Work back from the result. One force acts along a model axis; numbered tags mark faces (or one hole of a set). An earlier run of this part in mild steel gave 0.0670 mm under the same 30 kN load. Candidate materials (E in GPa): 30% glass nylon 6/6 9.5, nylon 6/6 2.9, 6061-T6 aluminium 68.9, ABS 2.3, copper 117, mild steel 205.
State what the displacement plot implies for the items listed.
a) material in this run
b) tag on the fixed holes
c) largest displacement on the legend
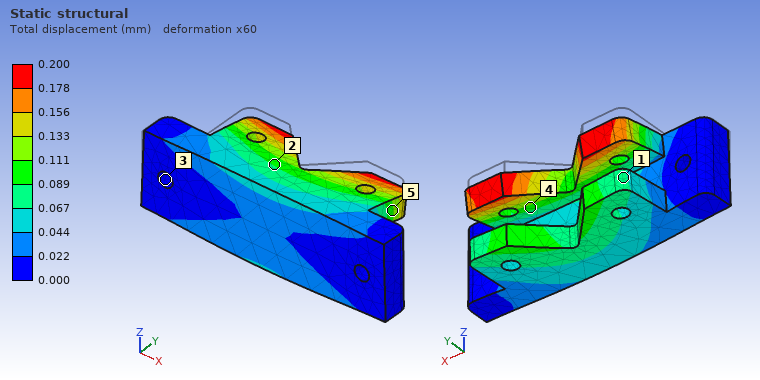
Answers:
6061-T6 aluminium
3
0.200 mm
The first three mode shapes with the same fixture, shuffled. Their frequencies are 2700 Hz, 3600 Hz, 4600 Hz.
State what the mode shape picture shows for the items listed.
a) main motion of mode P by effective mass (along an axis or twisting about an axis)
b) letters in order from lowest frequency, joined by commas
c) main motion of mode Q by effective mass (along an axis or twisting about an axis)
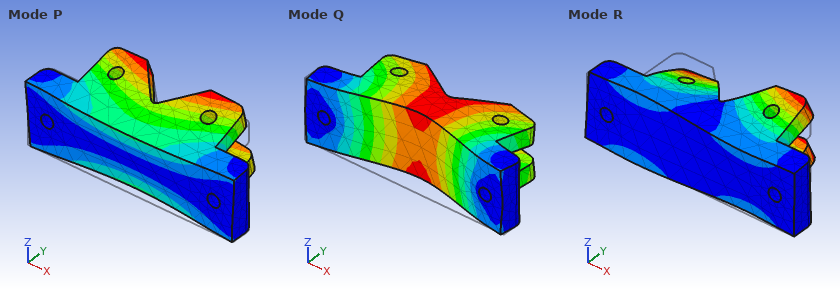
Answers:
along Z
P, Q, R
along Y
